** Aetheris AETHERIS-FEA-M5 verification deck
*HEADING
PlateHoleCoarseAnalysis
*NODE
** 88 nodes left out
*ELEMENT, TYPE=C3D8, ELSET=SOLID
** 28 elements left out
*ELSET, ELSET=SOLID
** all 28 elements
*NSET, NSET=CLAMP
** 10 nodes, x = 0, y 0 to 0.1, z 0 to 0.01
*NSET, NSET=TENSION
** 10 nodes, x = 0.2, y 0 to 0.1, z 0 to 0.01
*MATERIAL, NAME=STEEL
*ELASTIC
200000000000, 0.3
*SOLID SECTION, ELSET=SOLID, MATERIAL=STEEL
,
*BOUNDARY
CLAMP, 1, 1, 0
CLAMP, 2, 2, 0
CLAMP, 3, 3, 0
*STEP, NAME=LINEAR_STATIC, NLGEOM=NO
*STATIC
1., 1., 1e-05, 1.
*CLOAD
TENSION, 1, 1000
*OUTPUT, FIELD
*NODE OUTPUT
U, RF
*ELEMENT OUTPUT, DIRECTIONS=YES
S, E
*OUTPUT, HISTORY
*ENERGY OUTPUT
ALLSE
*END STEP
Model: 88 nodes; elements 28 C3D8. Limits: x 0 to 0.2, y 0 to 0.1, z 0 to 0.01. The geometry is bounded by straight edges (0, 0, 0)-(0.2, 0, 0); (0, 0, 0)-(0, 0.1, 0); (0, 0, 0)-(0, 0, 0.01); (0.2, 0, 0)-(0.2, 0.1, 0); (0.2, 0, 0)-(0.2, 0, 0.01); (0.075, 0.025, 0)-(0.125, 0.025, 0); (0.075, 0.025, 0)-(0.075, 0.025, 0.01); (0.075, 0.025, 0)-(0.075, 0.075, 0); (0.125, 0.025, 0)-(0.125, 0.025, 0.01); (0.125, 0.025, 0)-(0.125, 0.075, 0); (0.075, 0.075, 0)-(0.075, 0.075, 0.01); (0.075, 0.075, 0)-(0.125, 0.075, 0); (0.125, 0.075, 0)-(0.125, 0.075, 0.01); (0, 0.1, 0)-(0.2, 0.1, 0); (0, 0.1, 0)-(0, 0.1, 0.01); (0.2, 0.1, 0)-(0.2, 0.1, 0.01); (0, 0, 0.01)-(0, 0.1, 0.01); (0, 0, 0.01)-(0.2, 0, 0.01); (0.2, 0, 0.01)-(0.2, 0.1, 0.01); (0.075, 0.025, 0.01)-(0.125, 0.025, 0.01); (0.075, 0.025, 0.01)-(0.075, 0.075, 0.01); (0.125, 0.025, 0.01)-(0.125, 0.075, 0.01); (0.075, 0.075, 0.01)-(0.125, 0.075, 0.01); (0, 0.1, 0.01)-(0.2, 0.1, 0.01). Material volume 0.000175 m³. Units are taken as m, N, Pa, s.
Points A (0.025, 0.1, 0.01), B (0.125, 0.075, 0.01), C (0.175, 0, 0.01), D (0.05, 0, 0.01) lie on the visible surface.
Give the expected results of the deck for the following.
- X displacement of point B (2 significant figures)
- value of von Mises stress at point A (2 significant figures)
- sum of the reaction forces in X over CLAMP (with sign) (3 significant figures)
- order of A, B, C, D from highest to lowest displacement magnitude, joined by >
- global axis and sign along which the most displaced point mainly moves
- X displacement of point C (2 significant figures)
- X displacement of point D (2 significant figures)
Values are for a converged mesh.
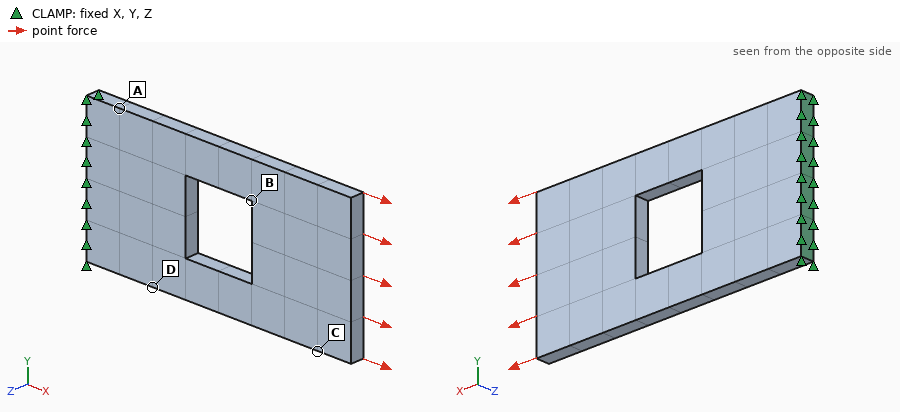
1.1e-05 m
1.3e+07 Pa
-10000 N
C > B > D > A
+X
1.4e-05 m
3.5e-06 m
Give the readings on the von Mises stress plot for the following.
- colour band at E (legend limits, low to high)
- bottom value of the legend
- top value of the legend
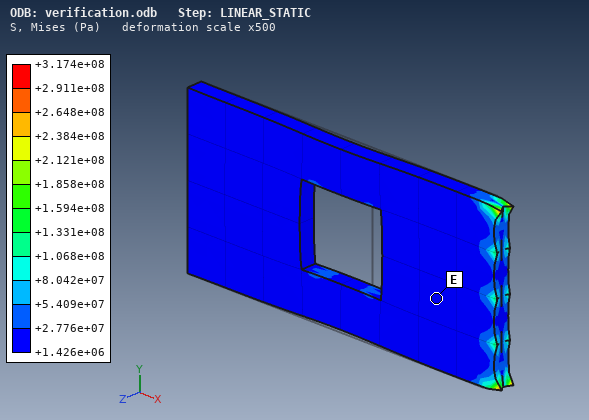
+1.426e+06 to +2.776e+07 Pa
+1.426e+06 Pa
+3.174e+08 Pa
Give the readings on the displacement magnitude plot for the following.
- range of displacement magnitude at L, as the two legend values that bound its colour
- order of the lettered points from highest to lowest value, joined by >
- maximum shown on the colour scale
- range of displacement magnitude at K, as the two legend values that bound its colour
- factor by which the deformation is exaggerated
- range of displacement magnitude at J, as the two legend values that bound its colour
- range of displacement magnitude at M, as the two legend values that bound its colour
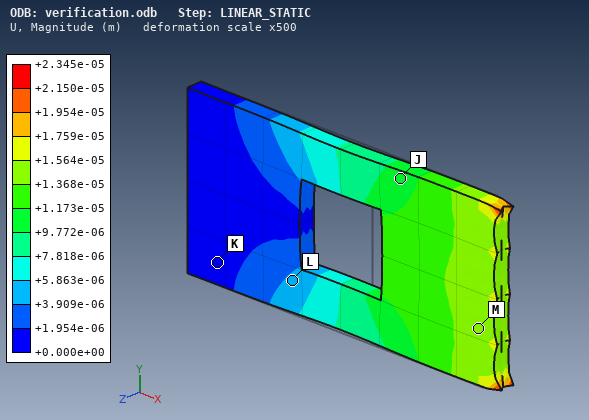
+3.909e-06 to +5.863e-06 m
M > J > L > K
+2.345e-05 m
+0.000e+00 to +1.954e-06 m
500
+9.772e-06 to +1.173e-05 m
+1.368e-05 to +1.564e-05 m
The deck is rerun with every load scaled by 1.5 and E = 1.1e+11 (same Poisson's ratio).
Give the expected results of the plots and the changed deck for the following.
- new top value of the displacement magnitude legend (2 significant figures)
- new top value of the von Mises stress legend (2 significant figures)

6.4e-05 m
4.8e+08 Pa
